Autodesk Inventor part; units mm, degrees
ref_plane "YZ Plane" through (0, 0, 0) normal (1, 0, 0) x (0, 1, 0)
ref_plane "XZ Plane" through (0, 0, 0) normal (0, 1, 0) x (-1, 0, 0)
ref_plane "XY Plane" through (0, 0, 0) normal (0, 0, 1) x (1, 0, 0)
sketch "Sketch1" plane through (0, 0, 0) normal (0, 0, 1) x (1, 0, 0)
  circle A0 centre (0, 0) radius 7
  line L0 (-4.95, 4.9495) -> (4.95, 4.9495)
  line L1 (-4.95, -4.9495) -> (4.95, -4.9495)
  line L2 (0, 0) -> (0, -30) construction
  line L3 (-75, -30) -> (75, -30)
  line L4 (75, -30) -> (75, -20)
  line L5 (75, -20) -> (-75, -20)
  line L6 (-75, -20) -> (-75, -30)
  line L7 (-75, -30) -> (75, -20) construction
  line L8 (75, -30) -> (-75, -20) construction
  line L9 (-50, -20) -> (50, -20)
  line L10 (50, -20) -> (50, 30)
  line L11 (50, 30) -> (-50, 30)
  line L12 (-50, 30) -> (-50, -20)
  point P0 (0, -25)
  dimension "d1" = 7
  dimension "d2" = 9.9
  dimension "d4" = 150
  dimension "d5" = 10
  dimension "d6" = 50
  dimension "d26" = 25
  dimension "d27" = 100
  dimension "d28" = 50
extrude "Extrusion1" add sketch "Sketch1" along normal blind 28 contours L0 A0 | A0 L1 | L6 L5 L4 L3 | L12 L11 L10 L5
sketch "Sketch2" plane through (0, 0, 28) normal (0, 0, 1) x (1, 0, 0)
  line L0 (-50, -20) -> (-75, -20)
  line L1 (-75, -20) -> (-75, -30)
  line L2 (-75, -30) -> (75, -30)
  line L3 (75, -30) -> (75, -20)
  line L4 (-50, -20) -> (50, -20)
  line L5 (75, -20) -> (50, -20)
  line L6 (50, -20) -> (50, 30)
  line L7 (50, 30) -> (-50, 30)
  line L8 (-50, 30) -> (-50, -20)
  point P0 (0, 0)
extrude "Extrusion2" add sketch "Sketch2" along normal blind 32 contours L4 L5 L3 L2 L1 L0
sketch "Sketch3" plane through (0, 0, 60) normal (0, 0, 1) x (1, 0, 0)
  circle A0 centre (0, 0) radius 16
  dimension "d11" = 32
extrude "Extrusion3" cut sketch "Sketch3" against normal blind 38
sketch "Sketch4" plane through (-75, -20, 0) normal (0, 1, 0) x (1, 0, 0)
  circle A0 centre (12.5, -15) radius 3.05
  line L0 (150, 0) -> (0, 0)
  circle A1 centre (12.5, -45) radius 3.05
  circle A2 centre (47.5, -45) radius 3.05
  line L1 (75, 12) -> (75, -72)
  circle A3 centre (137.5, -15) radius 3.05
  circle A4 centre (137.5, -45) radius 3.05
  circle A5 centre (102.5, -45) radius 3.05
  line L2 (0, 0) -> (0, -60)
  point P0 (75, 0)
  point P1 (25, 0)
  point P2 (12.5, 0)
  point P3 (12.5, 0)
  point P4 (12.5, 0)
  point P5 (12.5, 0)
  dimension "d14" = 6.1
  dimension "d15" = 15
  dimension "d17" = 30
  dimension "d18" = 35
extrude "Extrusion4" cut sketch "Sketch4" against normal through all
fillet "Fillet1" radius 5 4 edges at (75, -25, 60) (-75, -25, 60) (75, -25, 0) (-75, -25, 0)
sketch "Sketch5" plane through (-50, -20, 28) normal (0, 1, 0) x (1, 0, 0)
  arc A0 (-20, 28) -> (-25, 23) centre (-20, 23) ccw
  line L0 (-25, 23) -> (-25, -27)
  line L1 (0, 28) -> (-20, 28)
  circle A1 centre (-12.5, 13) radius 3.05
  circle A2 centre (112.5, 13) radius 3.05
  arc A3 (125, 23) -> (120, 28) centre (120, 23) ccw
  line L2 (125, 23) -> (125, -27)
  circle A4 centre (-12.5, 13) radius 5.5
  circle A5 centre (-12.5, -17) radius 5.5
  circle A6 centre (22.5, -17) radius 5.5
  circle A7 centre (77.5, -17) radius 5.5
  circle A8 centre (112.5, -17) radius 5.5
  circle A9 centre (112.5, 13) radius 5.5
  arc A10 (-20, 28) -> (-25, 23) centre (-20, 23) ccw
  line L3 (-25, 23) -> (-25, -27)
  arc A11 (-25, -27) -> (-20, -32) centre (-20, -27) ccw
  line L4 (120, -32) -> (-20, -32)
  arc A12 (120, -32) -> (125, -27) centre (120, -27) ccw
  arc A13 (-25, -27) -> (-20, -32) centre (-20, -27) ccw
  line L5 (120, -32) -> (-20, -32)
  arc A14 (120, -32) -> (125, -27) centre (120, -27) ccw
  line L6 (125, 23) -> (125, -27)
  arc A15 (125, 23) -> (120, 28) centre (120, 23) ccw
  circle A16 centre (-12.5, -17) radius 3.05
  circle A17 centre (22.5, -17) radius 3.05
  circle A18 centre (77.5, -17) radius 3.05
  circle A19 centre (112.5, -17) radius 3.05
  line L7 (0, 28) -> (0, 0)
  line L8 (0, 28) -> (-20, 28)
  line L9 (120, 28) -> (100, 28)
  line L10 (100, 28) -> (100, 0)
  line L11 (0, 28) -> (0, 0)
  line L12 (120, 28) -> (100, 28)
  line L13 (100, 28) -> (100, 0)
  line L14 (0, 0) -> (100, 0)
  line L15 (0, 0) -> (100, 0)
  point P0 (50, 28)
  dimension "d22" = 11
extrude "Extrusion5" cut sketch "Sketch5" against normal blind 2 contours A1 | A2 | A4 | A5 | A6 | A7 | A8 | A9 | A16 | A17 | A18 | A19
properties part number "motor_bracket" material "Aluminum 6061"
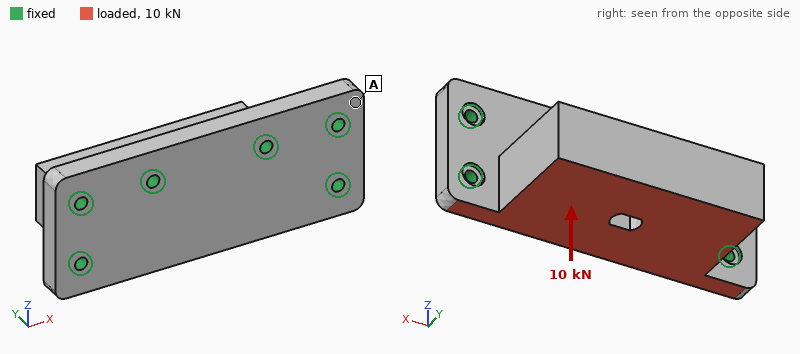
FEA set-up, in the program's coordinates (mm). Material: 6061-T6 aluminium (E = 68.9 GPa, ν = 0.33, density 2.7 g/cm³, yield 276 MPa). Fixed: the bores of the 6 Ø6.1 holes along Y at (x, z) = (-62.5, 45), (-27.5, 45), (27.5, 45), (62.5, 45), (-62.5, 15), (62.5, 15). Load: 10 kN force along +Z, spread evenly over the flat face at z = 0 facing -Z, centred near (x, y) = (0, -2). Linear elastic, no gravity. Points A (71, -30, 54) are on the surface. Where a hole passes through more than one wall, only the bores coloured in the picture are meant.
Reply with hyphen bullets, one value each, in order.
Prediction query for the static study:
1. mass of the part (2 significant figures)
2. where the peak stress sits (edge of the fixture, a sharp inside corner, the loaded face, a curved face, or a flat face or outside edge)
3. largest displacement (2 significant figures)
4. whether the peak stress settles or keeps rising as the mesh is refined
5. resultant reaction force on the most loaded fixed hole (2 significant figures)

- 590 g
- edge of the fixture
- 0.15 mm
- keeps rising
- 4.5 kN
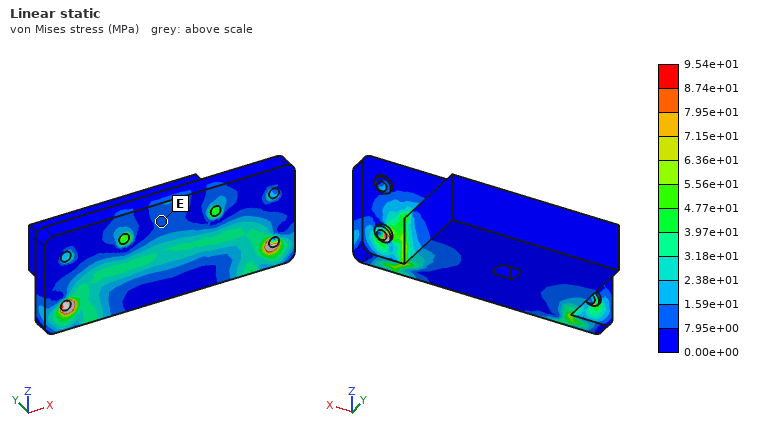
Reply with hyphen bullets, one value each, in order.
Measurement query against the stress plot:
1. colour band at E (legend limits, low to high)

- 7.95e+00 to 1.59e+01 MPa
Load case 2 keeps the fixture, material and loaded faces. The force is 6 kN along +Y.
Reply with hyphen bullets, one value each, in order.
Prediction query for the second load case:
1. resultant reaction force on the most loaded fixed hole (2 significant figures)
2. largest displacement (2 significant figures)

- 4.3 kN
- 98 µm
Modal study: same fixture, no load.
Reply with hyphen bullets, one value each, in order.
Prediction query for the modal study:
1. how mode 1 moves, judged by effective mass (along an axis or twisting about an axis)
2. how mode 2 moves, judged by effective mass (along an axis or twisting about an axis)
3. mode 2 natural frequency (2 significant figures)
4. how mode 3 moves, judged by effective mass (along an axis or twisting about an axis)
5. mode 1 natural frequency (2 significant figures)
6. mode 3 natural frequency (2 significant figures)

- along Z
- along X
- 5500 Hz
- along Y
- 2200 Hz
- 5800 Hz
